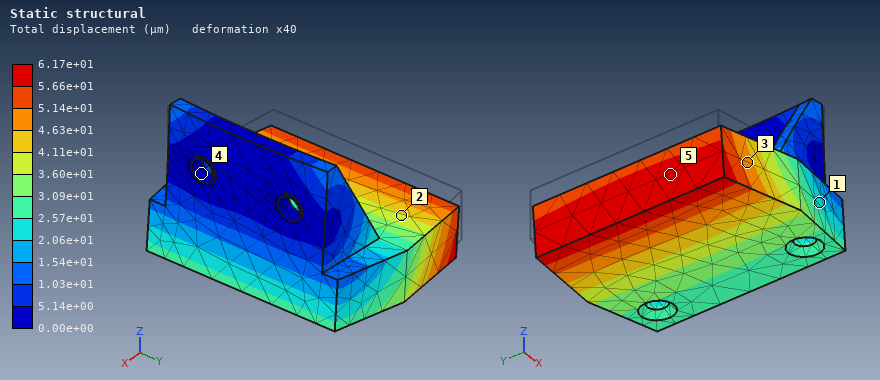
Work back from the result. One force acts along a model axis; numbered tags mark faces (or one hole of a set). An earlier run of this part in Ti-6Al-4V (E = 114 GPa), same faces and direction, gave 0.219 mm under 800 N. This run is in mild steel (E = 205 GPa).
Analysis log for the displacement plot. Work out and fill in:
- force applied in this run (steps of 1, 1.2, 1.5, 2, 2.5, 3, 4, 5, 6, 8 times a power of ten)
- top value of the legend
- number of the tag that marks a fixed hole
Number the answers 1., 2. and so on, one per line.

1. 400 N
2. 6.17e+01 µm
3. 4
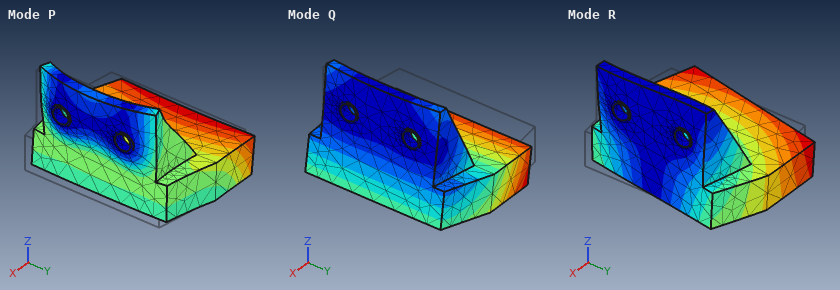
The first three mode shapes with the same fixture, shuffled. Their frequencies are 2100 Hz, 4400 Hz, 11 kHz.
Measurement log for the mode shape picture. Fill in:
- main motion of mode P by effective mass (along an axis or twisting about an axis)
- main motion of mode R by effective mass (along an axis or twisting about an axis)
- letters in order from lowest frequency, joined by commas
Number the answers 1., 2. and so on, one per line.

1. along X
2. along Y
3. Q, R, P
